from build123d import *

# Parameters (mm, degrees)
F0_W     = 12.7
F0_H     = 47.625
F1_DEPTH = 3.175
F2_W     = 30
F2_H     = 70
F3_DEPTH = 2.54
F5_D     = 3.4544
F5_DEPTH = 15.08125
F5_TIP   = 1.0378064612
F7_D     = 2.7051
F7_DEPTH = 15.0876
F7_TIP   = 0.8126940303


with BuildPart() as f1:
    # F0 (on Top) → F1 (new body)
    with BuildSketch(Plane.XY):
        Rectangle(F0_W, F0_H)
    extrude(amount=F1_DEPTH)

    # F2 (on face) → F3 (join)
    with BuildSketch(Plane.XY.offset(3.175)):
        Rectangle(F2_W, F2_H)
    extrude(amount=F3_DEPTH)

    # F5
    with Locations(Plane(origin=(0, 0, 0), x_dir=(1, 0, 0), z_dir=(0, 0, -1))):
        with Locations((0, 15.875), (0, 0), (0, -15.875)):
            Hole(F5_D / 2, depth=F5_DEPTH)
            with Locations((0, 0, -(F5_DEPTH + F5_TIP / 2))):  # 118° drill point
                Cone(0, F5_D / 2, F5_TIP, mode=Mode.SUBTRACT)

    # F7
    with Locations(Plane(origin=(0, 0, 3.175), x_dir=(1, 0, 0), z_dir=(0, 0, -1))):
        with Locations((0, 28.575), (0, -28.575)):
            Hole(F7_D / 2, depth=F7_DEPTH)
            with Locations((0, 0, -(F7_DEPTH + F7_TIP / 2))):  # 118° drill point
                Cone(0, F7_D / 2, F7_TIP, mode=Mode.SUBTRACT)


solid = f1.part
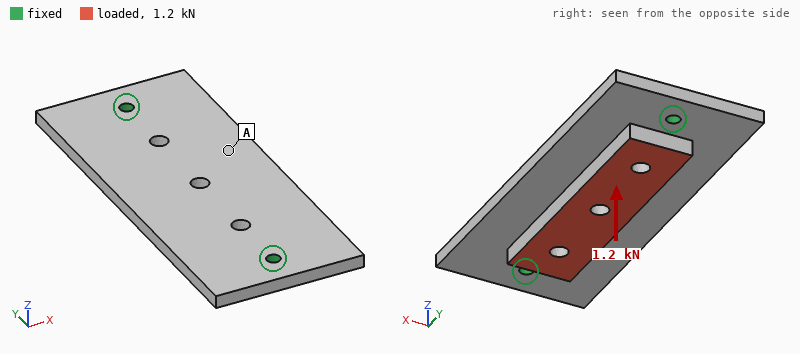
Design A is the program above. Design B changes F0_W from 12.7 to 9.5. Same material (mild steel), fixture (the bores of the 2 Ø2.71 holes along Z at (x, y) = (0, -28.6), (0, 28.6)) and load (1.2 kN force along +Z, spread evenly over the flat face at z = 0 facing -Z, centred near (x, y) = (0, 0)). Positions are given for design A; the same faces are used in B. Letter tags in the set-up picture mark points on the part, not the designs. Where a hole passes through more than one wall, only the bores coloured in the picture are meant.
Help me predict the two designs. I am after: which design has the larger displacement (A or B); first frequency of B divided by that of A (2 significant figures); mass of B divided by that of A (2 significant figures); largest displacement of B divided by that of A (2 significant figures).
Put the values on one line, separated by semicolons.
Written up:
B; 0.99; 0.93; 1.2
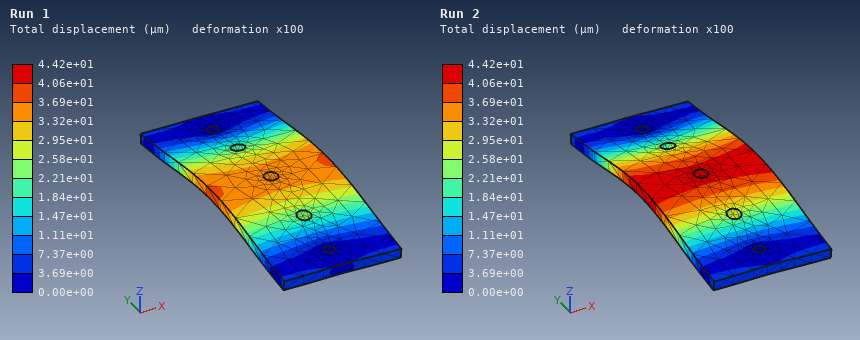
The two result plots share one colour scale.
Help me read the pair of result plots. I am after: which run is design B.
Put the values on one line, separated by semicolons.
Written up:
Run 2
